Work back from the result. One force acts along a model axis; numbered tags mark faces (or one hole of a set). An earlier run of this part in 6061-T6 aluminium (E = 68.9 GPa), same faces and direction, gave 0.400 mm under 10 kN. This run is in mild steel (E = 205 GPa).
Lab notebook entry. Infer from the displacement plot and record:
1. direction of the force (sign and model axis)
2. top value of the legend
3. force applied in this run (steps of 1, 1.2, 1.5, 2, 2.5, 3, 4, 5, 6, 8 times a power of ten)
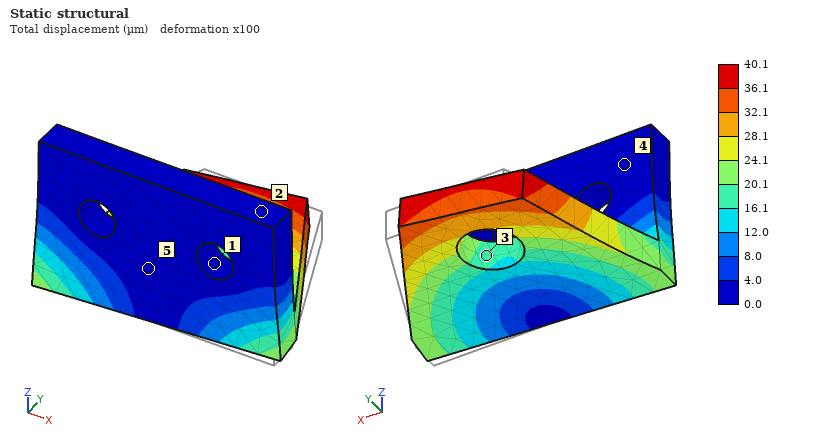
-X
40.1 µm
3 kN
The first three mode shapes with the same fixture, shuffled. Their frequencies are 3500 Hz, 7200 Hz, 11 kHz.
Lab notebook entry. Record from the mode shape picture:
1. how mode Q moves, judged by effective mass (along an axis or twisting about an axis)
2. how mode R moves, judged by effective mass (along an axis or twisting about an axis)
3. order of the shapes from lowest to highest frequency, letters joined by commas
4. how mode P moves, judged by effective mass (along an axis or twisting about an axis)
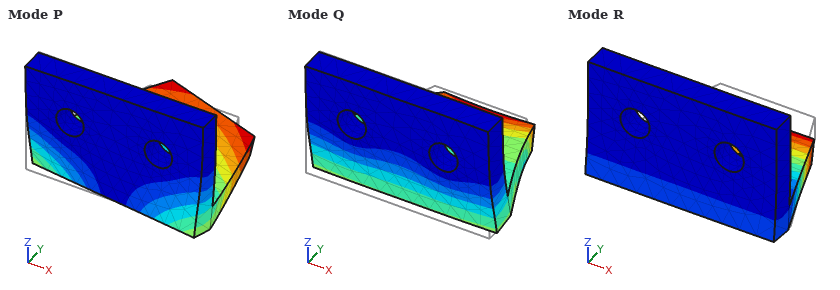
along Y
along Z
R, P, Q
along X
